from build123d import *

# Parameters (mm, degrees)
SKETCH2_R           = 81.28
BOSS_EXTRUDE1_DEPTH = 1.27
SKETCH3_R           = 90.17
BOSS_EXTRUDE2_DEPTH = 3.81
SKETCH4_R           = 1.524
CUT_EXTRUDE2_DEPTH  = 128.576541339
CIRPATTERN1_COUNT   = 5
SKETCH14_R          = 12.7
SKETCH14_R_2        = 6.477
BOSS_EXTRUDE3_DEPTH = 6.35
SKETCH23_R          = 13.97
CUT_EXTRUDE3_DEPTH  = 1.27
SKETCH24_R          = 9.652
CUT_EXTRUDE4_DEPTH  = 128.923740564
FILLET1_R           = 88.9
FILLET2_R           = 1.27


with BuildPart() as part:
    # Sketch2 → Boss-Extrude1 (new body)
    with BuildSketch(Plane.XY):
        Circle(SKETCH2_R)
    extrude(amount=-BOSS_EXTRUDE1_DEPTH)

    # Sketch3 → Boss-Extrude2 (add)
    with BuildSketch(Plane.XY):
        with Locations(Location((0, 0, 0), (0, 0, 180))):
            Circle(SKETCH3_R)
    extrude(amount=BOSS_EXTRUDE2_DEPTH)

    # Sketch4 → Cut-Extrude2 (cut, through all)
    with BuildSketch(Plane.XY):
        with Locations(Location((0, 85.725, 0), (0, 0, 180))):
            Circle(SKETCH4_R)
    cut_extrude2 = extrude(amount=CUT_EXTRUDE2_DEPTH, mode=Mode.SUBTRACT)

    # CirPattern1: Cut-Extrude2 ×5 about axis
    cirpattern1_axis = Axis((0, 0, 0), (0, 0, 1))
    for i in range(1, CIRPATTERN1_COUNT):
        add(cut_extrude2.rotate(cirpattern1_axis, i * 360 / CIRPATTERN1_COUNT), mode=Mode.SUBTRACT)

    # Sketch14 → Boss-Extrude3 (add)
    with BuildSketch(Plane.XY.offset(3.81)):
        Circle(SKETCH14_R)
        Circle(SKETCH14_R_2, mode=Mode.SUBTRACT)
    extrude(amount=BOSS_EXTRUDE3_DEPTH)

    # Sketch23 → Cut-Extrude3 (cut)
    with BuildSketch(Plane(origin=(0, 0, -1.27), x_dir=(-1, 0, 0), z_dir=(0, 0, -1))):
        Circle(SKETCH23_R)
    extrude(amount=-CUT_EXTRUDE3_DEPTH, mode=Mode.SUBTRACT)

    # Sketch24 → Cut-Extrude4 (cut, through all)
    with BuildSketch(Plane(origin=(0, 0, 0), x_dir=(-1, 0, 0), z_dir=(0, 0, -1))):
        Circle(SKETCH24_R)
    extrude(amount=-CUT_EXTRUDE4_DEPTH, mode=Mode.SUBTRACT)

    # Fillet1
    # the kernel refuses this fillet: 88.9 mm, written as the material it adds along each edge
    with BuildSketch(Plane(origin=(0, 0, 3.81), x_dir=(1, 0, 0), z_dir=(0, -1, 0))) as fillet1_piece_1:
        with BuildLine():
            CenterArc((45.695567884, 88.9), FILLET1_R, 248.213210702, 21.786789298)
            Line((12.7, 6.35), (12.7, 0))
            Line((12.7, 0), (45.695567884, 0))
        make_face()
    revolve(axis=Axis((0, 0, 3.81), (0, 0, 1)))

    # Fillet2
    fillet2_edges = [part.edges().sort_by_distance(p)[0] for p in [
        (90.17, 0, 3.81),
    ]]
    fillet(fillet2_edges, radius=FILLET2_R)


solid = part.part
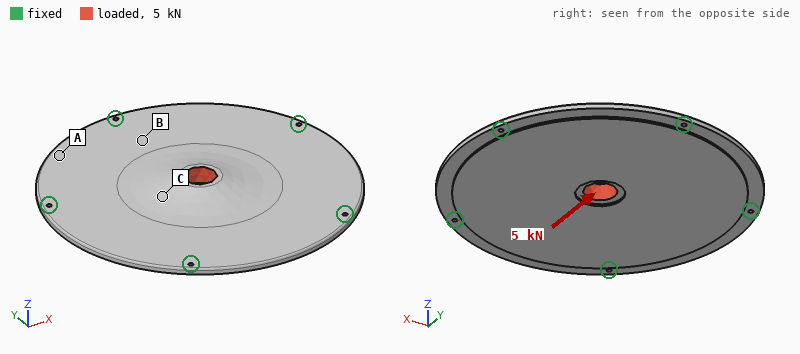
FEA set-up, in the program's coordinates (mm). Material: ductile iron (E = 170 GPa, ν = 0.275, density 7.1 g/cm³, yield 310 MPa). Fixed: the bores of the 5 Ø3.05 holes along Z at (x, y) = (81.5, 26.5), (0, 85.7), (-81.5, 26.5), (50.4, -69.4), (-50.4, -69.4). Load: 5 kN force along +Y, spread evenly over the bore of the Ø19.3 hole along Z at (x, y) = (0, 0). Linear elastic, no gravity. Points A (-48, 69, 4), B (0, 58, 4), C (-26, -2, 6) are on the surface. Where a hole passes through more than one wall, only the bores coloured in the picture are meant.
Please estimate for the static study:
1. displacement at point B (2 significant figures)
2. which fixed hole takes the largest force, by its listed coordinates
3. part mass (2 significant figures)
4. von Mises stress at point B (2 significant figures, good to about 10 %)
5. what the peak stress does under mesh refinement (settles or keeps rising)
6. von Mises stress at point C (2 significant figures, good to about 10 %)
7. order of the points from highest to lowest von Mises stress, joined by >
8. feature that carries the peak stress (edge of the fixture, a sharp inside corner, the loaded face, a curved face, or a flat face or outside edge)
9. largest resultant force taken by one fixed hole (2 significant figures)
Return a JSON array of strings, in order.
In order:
["9.7 µm", "(0, 85.7)", "940 g", "14 MPa", "keeps rising", "5.5 MPa", "B > C > A", "edge of the fixture", "1.2 kN"]
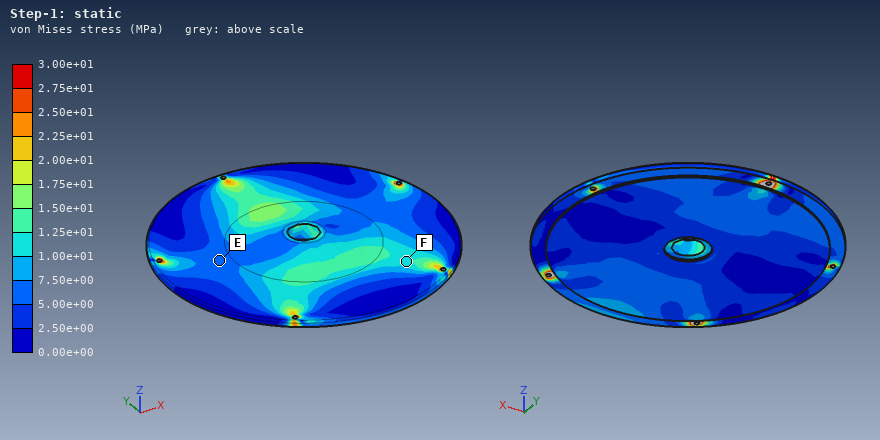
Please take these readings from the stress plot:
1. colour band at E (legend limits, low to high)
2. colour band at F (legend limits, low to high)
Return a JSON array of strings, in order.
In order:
["5.00e+00 to 7.50e+00 MPa", "1.00e+01 to 1.25e+01 MPa"]
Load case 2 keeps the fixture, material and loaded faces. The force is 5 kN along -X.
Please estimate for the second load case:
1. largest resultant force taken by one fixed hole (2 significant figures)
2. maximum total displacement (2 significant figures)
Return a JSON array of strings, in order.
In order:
["1.2 kN", "13 µm"]
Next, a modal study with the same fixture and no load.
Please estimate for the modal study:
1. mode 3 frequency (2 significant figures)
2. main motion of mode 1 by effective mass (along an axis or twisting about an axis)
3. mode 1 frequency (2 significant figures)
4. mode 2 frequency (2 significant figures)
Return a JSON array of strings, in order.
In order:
["1900 Hz", "along Z", "1100 Hz", "1900 Hz"]
